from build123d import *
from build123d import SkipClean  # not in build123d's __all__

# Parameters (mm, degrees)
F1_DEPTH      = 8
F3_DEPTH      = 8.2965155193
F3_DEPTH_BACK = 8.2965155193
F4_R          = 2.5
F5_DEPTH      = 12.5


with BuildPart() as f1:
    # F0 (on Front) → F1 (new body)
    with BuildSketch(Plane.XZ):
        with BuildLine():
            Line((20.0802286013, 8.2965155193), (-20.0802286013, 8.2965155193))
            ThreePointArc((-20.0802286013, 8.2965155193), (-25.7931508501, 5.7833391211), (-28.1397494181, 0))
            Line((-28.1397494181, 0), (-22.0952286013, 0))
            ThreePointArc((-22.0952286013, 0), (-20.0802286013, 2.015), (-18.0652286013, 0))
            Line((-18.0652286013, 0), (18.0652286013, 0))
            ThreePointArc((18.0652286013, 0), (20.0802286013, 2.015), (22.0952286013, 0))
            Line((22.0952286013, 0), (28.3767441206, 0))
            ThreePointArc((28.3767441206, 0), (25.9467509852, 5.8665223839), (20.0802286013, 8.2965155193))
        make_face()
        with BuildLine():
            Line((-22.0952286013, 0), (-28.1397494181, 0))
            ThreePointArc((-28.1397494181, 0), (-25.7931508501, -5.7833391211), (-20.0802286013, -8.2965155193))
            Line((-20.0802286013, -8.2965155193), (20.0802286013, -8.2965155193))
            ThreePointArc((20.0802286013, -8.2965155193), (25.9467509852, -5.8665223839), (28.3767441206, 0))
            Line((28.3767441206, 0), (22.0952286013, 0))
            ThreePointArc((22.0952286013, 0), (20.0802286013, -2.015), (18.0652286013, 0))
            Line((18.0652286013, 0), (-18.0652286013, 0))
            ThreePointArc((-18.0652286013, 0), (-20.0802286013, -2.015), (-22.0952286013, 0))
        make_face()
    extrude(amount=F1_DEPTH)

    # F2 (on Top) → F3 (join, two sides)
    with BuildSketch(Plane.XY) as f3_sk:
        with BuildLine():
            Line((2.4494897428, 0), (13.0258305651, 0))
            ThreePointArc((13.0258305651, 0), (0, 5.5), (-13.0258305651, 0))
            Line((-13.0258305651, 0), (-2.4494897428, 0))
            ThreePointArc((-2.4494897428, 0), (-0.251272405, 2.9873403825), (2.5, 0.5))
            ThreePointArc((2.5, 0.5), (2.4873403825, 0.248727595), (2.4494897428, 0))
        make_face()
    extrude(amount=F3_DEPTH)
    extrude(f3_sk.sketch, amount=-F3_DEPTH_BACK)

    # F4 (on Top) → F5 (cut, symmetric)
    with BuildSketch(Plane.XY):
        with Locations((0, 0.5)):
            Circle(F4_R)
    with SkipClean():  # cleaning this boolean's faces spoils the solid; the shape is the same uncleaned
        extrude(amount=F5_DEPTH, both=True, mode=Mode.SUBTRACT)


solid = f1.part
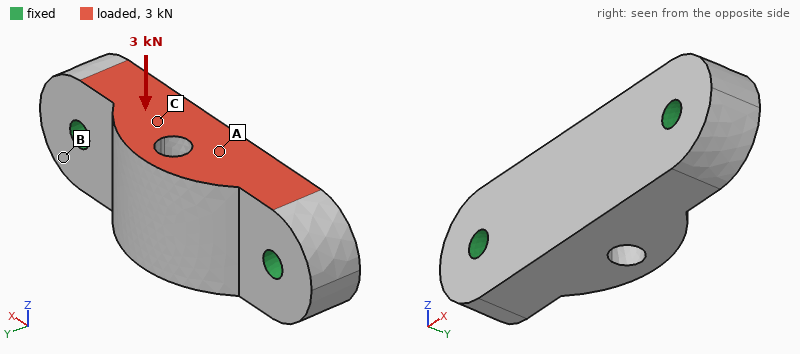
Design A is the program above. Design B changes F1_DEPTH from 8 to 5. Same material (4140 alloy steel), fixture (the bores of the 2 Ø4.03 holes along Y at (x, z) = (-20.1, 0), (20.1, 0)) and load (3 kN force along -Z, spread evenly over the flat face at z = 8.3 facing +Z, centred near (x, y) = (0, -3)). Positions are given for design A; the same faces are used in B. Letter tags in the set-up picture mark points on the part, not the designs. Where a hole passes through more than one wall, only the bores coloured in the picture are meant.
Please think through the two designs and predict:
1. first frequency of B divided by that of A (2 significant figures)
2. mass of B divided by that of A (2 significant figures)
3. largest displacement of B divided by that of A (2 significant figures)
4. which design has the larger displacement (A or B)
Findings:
0.81
0.69
1.9
B
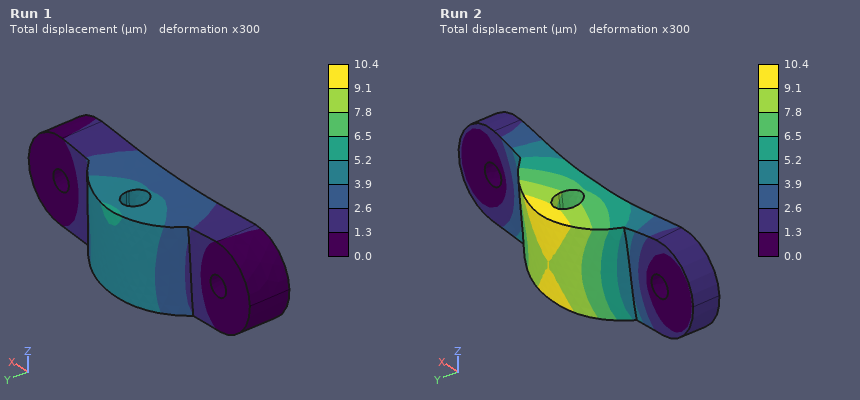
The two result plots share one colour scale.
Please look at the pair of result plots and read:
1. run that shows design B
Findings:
Run 2
